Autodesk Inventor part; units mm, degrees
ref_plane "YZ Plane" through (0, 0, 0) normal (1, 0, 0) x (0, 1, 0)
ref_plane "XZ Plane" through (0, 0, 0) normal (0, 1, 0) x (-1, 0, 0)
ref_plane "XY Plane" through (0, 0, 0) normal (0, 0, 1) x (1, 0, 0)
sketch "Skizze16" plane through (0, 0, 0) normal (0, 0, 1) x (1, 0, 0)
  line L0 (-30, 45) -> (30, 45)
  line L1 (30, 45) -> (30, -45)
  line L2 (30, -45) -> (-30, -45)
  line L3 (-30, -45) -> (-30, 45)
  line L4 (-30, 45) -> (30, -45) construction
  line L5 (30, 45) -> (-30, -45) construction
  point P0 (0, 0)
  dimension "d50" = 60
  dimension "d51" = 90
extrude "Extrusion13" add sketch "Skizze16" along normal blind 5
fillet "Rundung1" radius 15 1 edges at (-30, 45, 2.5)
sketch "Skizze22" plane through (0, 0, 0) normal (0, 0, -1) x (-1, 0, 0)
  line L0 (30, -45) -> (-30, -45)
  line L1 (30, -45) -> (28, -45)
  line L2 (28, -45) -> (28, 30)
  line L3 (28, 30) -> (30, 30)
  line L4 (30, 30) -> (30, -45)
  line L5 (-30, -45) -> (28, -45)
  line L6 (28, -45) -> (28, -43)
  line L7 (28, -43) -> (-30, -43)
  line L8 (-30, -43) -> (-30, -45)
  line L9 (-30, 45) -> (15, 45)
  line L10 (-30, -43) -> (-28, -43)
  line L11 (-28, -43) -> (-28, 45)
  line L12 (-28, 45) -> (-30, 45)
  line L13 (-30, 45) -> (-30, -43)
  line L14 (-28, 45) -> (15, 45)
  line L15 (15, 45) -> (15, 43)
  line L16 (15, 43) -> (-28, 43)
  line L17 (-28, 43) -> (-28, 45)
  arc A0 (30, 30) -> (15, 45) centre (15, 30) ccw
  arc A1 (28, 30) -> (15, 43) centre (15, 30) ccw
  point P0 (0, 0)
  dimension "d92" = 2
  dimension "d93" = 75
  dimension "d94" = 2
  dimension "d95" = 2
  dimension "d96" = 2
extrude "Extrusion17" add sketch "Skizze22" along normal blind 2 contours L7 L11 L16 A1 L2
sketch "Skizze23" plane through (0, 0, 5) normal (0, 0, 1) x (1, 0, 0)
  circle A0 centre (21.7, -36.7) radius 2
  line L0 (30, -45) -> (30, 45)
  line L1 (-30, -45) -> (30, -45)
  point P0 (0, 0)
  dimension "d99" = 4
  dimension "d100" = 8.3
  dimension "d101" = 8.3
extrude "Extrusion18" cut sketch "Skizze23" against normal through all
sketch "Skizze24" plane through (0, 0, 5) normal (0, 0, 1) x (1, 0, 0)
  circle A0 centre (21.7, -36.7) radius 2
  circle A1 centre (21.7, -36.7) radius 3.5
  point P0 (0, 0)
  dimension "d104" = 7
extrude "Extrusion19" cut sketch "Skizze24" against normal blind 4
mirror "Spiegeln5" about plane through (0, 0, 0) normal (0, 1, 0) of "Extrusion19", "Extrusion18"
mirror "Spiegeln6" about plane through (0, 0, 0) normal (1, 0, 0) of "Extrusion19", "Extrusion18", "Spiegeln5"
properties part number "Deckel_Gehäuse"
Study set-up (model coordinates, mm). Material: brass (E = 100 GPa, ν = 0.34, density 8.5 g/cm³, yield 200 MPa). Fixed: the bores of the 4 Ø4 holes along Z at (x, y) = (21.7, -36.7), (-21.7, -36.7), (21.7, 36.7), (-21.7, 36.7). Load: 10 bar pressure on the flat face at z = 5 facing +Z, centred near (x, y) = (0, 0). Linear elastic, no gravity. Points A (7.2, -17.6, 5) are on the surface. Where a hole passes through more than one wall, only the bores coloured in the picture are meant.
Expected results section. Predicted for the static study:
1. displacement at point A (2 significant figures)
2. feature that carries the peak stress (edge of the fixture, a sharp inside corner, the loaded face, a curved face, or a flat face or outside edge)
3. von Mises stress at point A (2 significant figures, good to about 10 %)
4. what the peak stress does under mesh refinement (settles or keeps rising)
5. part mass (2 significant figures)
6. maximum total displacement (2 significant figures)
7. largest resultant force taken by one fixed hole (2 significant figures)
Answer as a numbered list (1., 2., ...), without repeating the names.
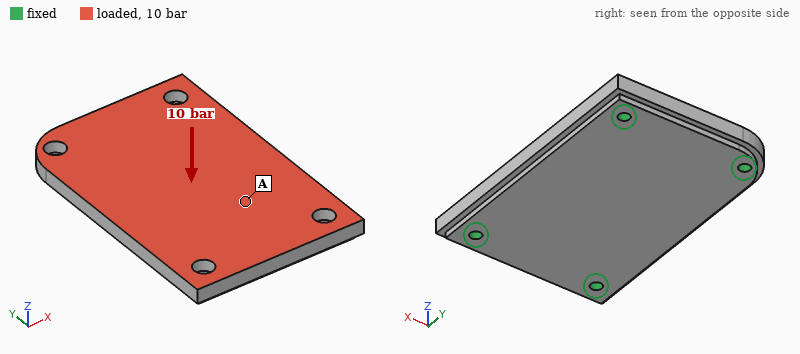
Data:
1. 46 µm
2. edge of the fixture
3. 26 MPa
4. keeps rising
5. 300 g
6. 64 µm
7. 1.9 kN
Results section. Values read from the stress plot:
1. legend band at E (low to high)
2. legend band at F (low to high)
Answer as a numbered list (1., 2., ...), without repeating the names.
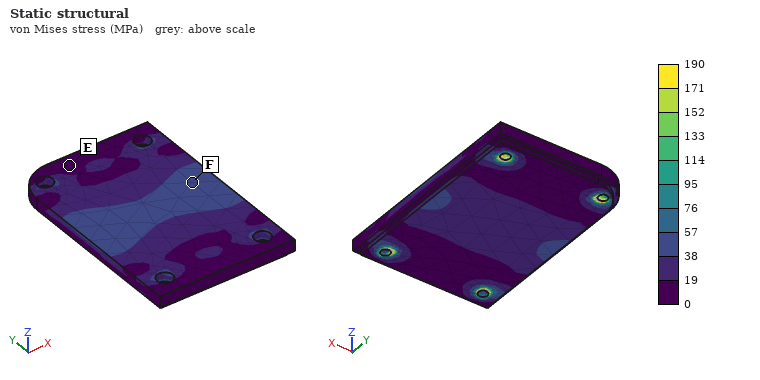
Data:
1. 0 to 19 MPa
2. 38 to 57 MPa
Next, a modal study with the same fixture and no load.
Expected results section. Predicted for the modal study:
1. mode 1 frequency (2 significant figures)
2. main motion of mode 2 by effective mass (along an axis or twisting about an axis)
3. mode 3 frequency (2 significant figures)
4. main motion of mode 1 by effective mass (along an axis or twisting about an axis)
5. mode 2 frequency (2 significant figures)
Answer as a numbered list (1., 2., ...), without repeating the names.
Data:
1. 2900 Hz
2. twisting about Y
3. 7600 Hz
4. along Z
5. 4600 Hz
